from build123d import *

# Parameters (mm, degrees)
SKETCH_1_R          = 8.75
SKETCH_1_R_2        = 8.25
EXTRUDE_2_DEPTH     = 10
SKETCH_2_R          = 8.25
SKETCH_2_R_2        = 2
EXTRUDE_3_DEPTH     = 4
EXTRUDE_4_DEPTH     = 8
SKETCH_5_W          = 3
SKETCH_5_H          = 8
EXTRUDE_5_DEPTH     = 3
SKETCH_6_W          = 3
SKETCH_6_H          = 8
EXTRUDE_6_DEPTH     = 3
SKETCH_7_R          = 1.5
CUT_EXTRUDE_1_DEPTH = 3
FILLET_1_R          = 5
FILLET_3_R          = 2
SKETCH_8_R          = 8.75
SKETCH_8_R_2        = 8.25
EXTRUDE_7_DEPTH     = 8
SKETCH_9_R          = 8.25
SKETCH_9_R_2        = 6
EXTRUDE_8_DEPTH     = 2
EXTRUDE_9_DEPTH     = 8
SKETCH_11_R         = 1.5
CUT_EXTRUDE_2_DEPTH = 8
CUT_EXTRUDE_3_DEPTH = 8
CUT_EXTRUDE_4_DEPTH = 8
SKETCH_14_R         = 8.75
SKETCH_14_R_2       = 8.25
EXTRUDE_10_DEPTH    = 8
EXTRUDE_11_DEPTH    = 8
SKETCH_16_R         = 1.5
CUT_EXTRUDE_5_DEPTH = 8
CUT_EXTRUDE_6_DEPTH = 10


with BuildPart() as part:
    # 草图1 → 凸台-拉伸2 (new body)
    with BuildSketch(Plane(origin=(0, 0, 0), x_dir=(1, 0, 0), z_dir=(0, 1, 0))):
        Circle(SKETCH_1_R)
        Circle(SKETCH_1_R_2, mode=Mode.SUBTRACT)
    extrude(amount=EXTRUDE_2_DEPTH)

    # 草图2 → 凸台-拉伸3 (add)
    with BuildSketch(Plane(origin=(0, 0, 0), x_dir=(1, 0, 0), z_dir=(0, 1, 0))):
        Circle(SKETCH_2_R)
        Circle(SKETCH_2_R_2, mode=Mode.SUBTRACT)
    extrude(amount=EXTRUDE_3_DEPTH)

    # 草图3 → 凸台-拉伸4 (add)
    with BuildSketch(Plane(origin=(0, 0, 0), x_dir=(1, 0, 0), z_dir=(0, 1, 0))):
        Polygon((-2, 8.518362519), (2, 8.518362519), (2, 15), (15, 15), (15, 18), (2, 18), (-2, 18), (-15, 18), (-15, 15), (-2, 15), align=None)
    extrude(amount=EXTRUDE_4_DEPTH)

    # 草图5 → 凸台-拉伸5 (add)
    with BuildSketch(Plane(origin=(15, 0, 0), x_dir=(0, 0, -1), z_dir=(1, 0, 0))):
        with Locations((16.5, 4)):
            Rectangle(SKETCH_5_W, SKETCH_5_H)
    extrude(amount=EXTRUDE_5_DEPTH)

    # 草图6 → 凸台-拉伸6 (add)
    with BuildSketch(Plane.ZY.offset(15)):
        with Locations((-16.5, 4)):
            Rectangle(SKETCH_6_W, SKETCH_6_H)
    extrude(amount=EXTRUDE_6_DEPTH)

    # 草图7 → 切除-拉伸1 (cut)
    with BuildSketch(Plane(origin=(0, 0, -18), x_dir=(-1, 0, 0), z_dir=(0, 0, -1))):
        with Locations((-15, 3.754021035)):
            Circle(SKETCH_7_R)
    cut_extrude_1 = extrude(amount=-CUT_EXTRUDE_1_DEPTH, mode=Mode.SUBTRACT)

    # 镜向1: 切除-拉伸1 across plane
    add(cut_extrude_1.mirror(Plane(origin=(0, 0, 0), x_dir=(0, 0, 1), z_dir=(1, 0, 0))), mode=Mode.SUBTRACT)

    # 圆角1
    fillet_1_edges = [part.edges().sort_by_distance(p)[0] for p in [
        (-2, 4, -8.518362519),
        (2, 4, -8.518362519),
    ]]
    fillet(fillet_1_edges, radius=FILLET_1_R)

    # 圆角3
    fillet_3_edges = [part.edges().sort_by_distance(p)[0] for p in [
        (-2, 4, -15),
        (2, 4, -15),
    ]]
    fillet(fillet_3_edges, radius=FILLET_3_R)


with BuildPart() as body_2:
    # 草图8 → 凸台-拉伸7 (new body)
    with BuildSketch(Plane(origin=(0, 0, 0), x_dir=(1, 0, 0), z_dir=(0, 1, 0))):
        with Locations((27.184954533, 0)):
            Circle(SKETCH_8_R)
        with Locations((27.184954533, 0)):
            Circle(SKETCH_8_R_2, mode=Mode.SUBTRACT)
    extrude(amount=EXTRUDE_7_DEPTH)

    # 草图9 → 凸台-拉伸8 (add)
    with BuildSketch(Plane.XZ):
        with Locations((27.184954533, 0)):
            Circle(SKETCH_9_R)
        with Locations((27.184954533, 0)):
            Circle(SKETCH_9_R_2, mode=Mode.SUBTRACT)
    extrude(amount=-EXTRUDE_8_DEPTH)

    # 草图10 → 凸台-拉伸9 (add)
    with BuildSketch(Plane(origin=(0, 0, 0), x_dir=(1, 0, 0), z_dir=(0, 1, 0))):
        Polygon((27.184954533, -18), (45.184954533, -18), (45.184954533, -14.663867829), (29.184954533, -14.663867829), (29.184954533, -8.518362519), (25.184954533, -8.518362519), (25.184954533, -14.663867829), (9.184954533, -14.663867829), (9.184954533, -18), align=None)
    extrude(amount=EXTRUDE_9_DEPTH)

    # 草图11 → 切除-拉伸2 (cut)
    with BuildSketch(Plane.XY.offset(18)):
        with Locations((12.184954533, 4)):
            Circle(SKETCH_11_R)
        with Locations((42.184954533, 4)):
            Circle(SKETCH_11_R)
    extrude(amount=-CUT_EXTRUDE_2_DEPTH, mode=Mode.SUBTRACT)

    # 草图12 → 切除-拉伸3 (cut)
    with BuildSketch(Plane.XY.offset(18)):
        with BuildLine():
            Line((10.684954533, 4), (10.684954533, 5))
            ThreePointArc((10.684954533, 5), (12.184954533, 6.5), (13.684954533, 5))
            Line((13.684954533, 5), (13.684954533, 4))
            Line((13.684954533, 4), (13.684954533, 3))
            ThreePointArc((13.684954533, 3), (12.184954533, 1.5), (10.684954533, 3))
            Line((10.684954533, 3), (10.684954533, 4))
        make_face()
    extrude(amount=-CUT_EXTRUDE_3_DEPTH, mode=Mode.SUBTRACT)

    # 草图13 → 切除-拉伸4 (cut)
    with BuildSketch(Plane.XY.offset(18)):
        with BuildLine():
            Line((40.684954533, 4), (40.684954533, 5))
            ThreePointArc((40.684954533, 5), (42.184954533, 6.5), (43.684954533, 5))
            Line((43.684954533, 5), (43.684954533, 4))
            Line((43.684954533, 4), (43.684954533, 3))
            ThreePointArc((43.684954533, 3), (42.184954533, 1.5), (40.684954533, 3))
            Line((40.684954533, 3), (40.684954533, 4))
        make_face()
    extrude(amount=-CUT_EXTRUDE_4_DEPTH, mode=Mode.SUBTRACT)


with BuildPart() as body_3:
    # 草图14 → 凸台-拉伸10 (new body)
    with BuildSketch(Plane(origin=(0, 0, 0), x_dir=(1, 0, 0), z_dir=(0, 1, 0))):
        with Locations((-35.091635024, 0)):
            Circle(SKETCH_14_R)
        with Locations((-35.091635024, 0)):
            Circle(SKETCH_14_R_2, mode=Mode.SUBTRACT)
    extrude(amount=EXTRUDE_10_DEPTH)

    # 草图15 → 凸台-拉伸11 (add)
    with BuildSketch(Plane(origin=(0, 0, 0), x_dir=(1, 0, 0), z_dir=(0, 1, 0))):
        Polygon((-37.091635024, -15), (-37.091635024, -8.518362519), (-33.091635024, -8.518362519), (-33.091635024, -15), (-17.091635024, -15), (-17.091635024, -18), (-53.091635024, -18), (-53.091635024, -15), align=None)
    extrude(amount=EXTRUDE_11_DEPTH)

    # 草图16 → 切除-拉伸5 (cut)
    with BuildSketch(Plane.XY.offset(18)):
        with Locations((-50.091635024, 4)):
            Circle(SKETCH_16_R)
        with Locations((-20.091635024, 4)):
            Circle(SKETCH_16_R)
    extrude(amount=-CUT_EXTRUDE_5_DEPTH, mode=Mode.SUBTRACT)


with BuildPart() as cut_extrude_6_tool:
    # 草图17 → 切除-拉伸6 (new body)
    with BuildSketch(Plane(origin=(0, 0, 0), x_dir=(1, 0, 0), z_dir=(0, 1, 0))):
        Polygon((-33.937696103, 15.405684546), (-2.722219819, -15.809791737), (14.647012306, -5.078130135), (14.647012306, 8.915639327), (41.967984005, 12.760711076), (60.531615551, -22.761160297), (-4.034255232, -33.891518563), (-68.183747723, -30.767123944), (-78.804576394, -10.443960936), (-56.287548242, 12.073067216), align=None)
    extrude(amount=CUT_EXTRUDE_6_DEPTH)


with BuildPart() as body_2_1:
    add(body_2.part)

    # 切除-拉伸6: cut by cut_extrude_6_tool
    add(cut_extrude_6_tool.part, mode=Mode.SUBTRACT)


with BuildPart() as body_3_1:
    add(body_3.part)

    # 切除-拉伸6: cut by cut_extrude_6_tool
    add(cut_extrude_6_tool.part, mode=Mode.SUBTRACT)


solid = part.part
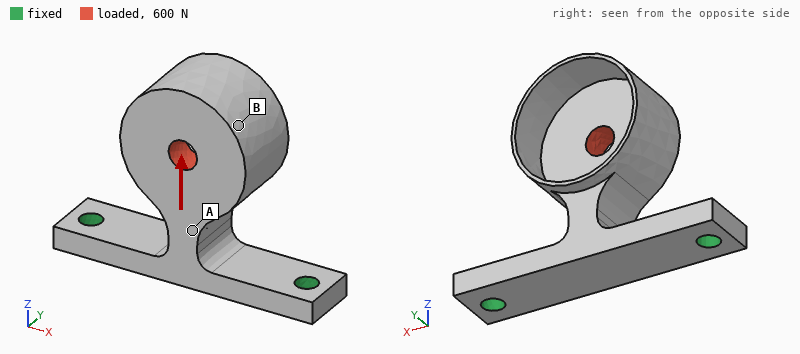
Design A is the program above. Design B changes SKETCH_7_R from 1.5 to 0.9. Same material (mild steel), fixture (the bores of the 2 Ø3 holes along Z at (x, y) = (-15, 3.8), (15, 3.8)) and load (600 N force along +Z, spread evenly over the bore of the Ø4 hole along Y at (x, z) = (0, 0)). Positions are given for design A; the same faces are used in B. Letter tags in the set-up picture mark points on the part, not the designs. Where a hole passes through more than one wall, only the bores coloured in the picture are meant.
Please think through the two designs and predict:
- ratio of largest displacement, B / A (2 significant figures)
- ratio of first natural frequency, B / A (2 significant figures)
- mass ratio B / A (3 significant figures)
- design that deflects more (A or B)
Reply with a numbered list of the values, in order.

1. 1.1
2. 0.95
3. 1.01
4. B
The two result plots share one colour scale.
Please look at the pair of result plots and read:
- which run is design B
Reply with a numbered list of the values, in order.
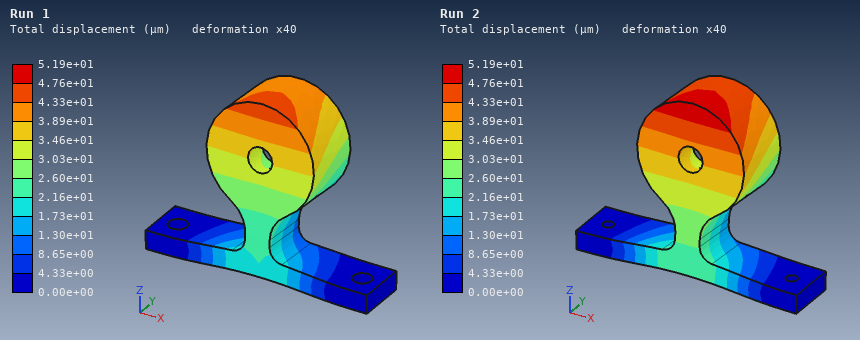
1. Run 2
